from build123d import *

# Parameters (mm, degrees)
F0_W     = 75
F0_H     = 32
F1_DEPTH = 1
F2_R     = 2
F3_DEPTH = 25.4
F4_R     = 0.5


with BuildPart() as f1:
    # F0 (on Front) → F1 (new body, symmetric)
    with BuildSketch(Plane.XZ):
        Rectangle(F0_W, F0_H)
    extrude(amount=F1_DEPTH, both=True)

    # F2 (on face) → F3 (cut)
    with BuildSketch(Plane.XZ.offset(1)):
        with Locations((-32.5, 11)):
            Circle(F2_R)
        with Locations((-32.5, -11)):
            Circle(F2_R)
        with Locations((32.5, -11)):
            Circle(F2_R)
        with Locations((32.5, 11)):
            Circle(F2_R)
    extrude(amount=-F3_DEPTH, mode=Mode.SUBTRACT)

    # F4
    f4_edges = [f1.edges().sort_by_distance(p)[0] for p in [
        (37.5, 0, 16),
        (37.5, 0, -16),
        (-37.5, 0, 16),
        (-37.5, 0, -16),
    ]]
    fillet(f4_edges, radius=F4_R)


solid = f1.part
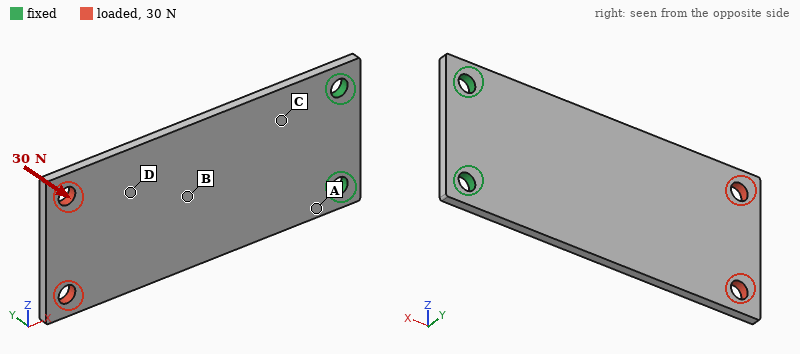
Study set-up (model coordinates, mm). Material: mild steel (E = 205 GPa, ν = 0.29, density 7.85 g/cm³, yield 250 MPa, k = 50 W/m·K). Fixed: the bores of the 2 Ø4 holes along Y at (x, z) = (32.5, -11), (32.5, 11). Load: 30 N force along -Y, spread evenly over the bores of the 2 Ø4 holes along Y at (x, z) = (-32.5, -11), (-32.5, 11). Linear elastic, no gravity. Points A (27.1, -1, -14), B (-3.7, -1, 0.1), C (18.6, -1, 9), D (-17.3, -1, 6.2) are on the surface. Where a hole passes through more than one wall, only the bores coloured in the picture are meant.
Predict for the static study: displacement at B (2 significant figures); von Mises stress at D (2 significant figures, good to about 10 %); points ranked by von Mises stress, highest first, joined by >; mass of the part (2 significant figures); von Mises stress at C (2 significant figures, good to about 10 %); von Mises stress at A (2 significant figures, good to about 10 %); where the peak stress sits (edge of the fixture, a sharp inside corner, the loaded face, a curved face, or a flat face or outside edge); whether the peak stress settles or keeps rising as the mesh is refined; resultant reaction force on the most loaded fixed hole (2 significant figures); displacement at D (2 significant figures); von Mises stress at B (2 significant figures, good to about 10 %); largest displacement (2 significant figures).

0.23 mm
22 MPa
A > C > B > D
37 g
68 MPa
93 MPa
edge of the fixture
keeps rising
15 N
0.40 mm
40 MPa
0.68 mm
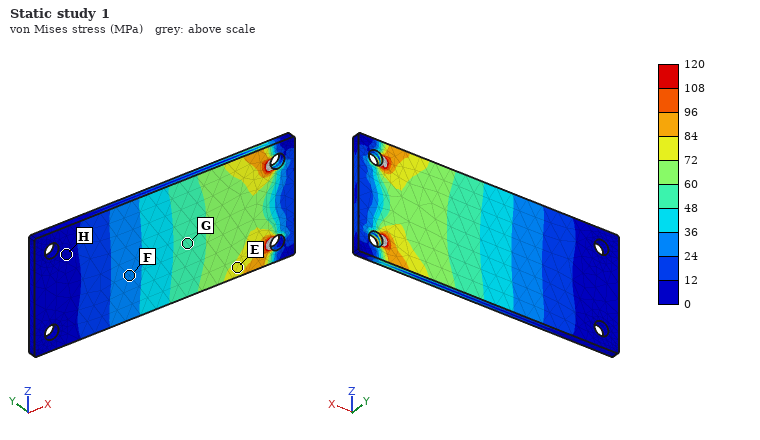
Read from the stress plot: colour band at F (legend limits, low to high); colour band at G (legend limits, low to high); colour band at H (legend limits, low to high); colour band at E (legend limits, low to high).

24 to 36 MPa
48 to 60 MPa
0 to 12 MPa
72 to 84 MPa
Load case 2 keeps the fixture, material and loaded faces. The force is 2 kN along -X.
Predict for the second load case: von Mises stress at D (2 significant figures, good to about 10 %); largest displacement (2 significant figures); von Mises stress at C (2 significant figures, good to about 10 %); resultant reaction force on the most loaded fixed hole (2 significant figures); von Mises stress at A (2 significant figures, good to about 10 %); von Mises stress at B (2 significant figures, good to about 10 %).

29 MPa
13 µm
32 MPa
1.0 kN
38 MPa
30 MPa
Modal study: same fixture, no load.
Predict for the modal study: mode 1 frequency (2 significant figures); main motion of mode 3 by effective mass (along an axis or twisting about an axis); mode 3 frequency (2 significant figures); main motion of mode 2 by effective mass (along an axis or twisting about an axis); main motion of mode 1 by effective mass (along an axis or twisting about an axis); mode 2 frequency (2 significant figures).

350 Hz
along Y
2200 Hz
twisting about X
along Y
1600 Hz
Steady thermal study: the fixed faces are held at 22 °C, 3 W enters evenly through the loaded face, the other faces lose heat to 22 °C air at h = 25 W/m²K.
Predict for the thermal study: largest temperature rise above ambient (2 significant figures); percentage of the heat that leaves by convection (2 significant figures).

37 K
62 %
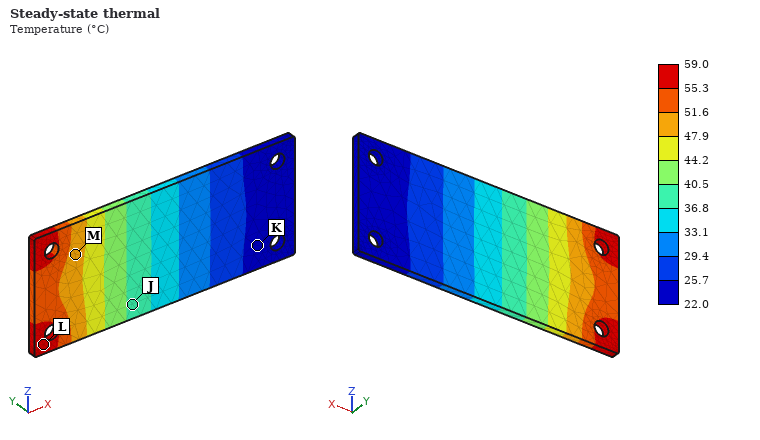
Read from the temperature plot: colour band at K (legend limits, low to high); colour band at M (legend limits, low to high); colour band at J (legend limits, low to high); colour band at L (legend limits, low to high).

22.0 to 25.7 °C
47.9 to 51.6 °C
36.8 to 40.5 °C
55.3 to 59.0 °C
